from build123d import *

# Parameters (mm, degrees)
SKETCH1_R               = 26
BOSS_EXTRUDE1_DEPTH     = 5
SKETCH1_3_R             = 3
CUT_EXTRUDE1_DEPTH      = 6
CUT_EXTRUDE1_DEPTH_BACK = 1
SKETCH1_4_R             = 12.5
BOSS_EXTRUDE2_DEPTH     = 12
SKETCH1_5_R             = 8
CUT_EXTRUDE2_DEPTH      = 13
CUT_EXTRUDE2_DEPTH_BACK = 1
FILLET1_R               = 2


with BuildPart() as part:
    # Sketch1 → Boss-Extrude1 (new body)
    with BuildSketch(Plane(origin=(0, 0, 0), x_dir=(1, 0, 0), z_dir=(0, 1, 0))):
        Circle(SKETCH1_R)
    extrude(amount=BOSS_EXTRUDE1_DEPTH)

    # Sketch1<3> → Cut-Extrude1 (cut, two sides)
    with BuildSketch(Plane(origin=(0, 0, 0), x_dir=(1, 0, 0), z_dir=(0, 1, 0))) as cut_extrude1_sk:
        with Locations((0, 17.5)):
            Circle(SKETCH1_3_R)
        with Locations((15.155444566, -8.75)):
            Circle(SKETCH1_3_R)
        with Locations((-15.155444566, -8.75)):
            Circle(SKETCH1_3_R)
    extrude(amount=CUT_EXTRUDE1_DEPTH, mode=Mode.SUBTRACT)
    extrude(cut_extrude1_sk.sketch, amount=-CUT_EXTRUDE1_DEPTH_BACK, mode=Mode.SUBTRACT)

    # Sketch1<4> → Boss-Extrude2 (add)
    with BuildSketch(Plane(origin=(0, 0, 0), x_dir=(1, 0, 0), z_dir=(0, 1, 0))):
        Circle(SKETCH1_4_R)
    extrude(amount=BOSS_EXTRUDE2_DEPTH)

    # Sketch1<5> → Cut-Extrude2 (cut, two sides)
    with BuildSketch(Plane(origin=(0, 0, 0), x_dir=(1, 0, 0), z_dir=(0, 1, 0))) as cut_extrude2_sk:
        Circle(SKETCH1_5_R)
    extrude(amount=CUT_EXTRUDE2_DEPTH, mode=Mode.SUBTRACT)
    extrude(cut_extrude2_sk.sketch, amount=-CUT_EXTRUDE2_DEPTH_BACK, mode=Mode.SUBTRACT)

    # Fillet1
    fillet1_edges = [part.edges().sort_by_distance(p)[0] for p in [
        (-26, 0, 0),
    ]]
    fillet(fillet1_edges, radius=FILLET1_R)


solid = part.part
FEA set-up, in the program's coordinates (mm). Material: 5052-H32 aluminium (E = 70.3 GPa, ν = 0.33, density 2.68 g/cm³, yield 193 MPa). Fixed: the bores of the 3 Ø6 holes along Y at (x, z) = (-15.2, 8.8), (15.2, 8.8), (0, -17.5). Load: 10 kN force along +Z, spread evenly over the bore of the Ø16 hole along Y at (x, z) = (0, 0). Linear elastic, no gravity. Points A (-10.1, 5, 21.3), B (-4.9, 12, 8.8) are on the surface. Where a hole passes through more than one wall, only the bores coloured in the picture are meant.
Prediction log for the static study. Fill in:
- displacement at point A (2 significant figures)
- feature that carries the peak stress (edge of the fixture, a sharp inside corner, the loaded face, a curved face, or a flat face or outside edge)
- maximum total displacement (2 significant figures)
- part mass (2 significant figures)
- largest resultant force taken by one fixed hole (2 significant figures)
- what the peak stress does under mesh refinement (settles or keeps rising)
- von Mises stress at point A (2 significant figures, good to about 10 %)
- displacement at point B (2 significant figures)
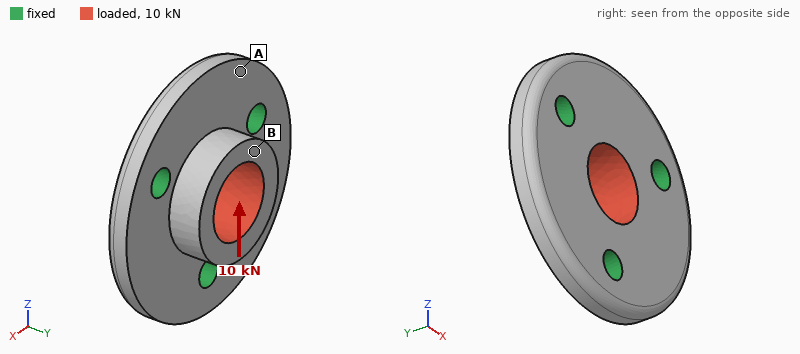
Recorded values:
9.9 µm
edge of the fixture
26 µm
30 g
3.5 kN
keeps rising
15 MPa
22 µm
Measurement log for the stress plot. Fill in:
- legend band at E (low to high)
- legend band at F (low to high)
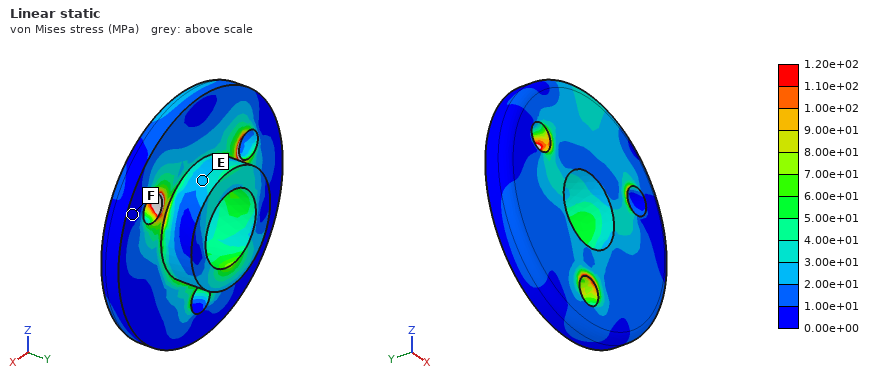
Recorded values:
2.00e+01 to 3.00e+01 MPa
0.00e+00 to 1.00e+01 MPa
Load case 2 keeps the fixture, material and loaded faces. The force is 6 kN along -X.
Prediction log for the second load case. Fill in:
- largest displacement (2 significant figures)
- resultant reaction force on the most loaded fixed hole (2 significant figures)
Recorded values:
14 µm
2.1 kN
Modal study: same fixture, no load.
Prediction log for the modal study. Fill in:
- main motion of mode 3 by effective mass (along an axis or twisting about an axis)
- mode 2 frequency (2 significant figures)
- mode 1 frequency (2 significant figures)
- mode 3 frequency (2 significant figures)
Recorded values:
along Y
16 kHz
16 kHz
18 kHz
